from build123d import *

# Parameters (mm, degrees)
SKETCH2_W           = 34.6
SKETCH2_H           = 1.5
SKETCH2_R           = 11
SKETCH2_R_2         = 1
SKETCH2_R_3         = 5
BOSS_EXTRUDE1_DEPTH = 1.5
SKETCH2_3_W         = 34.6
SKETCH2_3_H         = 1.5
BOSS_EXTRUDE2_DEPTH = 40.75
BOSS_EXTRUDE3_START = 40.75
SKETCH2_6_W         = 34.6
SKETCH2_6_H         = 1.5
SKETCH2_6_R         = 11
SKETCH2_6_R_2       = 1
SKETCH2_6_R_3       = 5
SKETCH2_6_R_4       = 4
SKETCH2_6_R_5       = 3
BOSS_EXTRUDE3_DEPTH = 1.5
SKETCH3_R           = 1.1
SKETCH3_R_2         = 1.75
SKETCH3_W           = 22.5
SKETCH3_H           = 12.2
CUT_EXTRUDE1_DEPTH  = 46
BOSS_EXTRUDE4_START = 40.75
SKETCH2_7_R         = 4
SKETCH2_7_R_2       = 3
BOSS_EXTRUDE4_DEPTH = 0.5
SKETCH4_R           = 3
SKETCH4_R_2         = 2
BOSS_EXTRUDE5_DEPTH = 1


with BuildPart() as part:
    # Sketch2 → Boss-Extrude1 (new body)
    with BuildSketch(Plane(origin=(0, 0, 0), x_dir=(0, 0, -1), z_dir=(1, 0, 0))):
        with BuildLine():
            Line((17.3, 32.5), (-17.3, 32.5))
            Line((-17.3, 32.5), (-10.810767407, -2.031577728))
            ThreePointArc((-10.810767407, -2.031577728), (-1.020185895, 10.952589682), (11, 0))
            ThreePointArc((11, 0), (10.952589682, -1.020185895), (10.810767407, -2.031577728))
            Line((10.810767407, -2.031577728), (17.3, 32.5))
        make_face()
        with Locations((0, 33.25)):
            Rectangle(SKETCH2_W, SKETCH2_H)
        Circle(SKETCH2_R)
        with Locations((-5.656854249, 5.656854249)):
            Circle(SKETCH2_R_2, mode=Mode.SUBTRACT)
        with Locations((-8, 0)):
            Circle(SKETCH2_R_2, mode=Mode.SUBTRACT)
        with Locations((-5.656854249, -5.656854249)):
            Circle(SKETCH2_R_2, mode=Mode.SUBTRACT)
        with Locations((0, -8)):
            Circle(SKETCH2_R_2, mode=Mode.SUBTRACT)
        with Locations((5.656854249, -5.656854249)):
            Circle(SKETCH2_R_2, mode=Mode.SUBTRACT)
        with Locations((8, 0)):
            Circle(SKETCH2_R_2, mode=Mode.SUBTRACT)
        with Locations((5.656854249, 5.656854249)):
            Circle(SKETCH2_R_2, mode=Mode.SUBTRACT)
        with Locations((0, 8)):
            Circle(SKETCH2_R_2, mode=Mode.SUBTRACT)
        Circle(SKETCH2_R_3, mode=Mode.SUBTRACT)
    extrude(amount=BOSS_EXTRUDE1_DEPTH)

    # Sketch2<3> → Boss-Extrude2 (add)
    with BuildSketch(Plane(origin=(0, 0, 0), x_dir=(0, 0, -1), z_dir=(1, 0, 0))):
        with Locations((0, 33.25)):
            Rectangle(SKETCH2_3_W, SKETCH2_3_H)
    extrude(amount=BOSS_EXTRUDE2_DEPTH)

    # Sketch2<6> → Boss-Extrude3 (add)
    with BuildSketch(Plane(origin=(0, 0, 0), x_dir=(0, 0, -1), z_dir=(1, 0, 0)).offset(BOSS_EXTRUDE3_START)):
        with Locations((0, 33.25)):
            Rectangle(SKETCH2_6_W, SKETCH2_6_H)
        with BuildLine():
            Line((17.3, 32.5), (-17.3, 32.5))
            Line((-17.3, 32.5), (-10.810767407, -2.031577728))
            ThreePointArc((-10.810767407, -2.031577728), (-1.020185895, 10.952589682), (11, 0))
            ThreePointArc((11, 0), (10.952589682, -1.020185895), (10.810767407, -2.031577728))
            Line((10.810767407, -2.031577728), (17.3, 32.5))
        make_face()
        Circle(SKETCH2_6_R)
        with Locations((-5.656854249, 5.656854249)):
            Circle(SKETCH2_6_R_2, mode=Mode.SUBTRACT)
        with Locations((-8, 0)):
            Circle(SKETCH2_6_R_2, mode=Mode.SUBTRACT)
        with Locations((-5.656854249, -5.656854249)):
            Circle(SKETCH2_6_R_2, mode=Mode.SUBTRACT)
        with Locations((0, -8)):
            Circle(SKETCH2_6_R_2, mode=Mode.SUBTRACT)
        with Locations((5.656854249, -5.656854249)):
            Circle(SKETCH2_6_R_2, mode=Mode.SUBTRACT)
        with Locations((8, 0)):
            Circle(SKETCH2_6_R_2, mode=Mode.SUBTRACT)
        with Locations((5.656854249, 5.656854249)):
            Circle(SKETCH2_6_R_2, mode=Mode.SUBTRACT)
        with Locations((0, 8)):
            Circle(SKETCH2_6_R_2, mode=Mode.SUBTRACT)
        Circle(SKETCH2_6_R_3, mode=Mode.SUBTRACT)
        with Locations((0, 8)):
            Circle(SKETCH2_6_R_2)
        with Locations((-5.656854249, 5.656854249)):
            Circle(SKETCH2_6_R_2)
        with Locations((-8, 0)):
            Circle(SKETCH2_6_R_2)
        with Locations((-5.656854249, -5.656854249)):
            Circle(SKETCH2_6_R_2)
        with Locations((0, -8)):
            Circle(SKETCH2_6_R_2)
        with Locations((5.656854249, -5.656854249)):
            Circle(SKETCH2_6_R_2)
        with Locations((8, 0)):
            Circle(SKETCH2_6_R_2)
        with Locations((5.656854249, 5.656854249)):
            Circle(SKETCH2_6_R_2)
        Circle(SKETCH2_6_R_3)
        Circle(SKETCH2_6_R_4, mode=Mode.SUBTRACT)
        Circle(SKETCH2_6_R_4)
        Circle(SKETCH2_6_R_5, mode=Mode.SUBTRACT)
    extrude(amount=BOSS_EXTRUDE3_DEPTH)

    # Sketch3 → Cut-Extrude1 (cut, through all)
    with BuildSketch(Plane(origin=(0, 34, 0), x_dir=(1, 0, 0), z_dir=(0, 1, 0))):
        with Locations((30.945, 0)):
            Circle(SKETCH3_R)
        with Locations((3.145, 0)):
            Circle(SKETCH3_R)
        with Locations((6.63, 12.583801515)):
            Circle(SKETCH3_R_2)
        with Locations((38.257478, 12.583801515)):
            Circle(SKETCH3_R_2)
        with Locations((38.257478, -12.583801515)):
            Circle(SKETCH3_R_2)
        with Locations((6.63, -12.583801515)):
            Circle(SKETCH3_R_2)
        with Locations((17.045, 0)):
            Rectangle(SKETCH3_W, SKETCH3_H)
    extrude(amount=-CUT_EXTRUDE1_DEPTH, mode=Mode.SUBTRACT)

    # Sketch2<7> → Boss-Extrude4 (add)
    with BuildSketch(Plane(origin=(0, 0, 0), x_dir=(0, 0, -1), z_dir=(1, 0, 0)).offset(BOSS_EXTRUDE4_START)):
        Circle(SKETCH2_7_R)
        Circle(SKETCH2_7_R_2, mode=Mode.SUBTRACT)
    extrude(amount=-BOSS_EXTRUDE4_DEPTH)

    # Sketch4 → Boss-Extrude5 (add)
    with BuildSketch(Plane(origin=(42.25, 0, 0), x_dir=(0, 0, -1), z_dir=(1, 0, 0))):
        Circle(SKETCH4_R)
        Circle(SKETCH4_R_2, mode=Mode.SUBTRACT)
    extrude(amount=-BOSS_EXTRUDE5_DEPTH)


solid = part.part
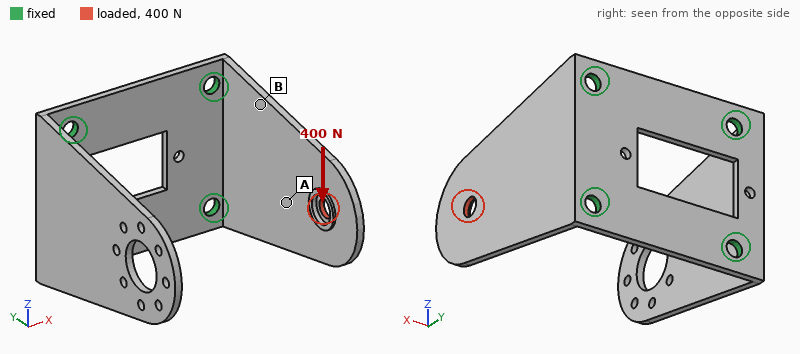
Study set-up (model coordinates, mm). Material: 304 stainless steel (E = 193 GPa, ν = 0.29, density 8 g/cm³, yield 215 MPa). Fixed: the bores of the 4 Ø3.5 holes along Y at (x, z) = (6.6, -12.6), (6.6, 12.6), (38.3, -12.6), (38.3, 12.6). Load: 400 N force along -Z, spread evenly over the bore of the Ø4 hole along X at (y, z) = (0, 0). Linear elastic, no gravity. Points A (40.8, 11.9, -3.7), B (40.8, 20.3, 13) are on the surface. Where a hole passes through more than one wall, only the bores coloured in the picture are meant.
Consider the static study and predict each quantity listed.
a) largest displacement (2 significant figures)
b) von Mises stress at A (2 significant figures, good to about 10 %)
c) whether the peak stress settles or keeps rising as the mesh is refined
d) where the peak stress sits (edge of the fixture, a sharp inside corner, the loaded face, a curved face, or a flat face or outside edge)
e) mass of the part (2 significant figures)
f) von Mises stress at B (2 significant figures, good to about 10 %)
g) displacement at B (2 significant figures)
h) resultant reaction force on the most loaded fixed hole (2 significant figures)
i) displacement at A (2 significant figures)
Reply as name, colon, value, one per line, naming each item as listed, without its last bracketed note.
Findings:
largest displacement: 29 µm
von Mises stress at A: 16 MPa
whether the peak stress settles or keeps rising as the mesh is refined: keeps rising
where the peak stress sits: edge of the fixture
mass of the part: 39 g
von Mises stress at B: 43 MPa
displacement at B: 13 µm
resultant reaction force on the most loaded fixed hole: 560 N
displacement at A: 13 µm
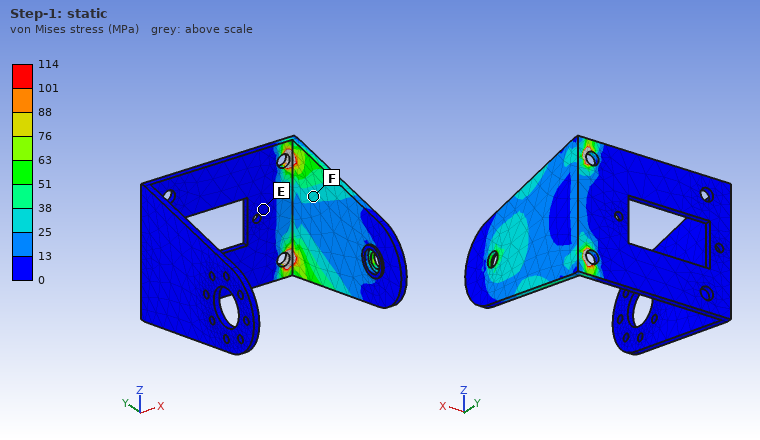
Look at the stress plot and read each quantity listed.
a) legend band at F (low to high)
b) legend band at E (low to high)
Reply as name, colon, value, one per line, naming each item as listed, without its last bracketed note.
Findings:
legend band at F: 25 to 38 MPa
legend band at E: 0 to 13 MPa
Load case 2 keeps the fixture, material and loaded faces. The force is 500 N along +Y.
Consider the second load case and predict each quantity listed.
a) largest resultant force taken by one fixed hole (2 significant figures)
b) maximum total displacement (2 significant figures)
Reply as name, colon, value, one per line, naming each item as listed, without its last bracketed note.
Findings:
largest resultant force taken by one fixed hole: 260 N
maximum total displacement: 0.12 mm
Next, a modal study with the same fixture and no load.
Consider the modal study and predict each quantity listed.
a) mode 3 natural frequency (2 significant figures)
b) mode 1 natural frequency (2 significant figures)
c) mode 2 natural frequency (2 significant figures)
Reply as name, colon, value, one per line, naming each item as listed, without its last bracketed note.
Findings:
mode 3 natural frequency: 2900 Hz
mode 1 natural frequency: 720 Hz
mode 2 natural frequency: 730 Hz
